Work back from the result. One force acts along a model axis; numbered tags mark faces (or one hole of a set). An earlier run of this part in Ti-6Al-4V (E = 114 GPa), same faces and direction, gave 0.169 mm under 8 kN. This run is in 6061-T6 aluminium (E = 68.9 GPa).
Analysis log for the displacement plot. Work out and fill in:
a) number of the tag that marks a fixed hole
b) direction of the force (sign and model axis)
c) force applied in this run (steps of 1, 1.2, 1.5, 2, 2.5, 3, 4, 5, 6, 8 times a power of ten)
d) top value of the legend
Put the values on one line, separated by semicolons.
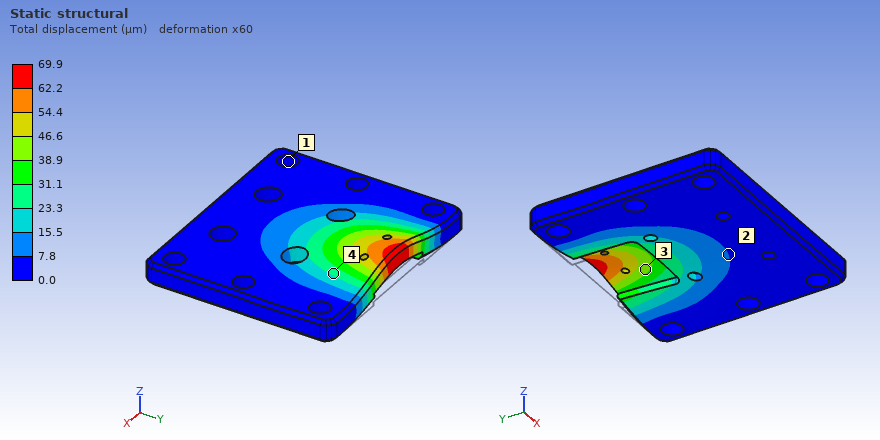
1; +Z; 2 kN; 69.9 µm
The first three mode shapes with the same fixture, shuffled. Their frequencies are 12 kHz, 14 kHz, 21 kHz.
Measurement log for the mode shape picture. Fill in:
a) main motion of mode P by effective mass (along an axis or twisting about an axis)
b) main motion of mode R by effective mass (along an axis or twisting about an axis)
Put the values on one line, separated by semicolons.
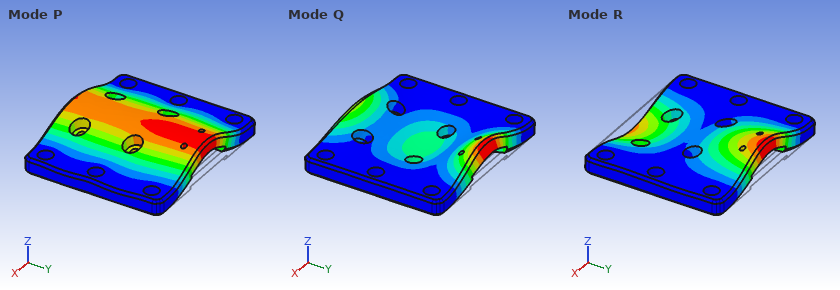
along Z; twisting about X
